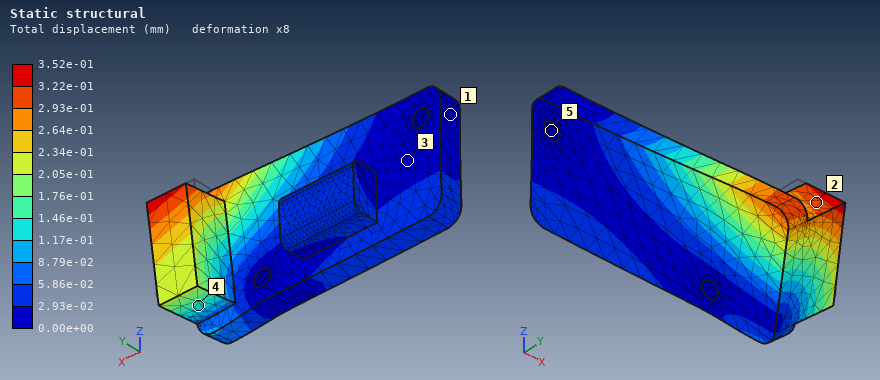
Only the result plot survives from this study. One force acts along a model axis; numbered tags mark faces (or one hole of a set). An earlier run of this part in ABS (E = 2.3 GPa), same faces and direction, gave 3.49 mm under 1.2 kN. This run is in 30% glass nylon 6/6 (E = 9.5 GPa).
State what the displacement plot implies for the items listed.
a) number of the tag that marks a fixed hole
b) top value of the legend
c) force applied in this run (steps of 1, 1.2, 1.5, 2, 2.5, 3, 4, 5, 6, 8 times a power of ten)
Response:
5
3.52e-01 mm
500 N
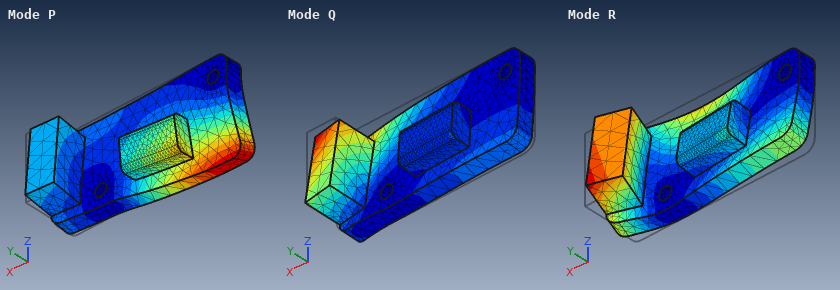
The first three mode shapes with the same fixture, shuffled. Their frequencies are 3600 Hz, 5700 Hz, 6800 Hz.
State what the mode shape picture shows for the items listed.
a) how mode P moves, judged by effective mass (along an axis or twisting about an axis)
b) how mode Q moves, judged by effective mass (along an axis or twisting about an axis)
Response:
along Y
along Y
